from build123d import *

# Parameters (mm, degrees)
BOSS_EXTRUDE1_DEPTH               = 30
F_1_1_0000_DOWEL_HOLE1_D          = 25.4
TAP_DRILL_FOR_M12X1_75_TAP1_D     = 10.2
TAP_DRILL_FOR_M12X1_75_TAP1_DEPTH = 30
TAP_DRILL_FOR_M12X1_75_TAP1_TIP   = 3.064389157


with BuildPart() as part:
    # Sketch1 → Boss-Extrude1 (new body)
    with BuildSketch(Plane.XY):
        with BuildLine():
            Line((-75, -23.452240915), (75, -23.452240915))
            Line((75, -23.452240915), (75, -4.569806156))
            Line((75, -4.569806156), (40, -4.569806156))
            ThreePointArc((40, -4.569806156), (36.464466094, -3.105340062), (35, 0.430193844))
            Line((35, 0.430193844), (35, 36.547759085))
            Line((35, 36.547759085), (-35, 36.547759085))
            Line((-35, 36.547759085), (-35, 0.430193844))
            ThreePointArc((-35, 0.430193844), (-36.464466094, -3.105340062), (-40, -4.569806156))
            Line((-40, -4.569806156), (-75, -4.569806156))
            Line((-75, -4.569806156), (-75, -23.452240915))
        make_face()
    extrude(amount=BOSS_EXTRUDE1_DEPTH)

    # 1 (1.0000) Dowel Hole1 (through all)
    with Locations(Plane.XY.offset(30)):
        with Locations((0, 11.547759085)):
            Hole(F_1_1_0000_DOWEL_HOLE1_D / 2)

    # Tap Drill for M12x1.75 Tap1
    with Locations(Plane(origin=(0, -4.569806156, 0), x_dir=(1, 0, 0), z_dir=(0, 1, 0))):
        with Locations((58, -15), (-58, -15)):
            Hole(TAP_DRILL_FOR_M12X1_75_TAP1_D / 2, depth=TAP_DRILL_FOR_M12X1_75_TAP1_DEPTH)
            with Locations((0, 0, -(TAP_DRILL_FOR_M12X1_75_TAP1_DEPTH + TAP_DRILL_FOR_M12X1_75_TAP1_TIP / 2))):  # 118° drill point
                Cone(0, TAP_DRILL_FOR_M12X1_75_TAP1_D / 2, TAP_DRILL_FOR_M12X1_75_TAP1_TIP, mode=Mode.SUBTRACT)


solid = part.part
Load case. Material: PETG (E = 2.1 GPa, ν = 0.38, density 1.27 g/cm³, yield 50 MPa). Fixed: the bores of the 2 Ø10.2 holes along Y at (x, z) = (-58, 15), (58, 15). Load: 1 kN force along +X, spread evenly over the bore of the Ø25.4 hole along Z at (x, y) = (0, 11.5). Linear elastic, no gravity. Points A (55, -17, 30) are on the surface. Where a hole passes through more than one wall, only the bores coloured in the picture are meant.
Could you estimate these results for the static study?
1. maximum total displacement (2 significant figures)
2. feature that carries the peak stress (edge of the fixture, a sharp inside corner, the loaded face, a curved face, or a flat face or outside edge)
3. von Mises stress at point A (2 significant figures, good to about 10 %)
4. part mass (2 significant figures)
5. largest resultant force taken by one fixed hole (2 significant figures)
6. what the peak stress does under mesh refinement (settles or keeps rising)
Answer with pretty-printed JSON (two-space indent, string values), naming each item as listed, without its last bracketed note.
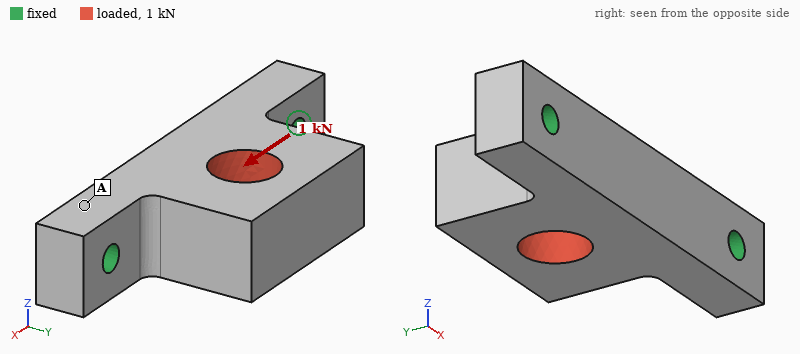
{
  "maximum total displacement": "75 µm",
  "feature that carries the peak stress": "edge of the fixture",
  "von Mises stress at point A": "0.59 MPa",
  "part mass": "190 g",
  "largest resultant force taken by one fixed hole": "570 N",
  "what the peak stress does under mesh refinement": "keeps rising"
}
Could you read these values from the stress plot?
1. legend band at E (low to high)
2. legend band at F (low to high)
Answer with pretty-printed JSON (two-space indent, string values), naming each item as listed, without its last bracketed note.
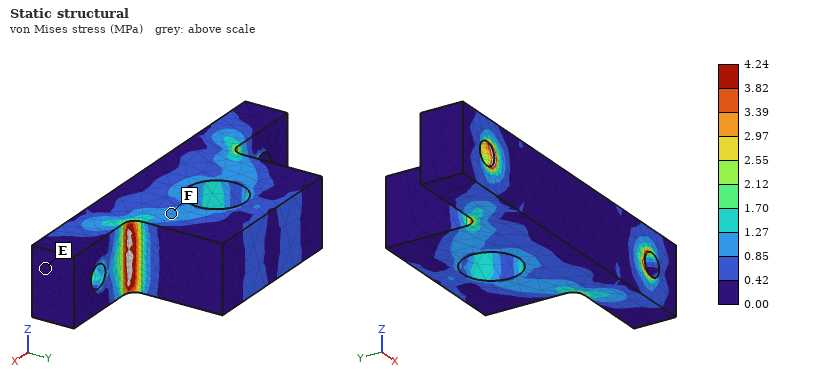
{
  "legend band at E": "0.00 to 0.42 MPa",
  "legend band at F": "0.85 to 1.27 MPa"
}
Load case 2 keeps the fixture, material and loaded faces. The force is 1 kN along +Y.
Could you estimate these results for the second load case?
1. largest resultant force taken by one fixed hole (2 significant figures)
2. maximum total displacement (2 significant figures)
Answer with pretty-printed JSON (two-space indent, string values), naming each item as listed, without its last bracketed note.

{
  "largest resultant force taken by one fixed hole": "550 N",
  "maximum total displacement": "92 µm"
}
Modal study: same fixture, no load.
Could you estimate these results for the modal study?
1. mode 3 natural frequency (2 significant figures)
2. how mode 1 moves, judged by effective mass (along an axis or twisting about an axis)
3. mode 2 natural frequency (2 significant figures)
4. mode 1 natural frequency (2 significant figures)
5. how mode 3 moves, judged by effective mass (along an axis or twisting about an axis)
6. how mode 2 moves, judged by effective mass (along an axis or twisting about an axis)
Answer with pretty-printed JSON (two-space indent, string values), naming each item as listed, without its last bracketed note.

{
  "mode 3 natural frequency": "1900 Hz",
  "how mode 1 moves, judged by effective mass": "along Z",
  "mode 2 natural frequency": "1500 Hz",
  "mode 1 natural frequency": "670 Hz",
  "how mode 3 moves, judged by effective mass": "along Z",
  "how mode 2 moves, judged by effective mass": "along Y"
}
